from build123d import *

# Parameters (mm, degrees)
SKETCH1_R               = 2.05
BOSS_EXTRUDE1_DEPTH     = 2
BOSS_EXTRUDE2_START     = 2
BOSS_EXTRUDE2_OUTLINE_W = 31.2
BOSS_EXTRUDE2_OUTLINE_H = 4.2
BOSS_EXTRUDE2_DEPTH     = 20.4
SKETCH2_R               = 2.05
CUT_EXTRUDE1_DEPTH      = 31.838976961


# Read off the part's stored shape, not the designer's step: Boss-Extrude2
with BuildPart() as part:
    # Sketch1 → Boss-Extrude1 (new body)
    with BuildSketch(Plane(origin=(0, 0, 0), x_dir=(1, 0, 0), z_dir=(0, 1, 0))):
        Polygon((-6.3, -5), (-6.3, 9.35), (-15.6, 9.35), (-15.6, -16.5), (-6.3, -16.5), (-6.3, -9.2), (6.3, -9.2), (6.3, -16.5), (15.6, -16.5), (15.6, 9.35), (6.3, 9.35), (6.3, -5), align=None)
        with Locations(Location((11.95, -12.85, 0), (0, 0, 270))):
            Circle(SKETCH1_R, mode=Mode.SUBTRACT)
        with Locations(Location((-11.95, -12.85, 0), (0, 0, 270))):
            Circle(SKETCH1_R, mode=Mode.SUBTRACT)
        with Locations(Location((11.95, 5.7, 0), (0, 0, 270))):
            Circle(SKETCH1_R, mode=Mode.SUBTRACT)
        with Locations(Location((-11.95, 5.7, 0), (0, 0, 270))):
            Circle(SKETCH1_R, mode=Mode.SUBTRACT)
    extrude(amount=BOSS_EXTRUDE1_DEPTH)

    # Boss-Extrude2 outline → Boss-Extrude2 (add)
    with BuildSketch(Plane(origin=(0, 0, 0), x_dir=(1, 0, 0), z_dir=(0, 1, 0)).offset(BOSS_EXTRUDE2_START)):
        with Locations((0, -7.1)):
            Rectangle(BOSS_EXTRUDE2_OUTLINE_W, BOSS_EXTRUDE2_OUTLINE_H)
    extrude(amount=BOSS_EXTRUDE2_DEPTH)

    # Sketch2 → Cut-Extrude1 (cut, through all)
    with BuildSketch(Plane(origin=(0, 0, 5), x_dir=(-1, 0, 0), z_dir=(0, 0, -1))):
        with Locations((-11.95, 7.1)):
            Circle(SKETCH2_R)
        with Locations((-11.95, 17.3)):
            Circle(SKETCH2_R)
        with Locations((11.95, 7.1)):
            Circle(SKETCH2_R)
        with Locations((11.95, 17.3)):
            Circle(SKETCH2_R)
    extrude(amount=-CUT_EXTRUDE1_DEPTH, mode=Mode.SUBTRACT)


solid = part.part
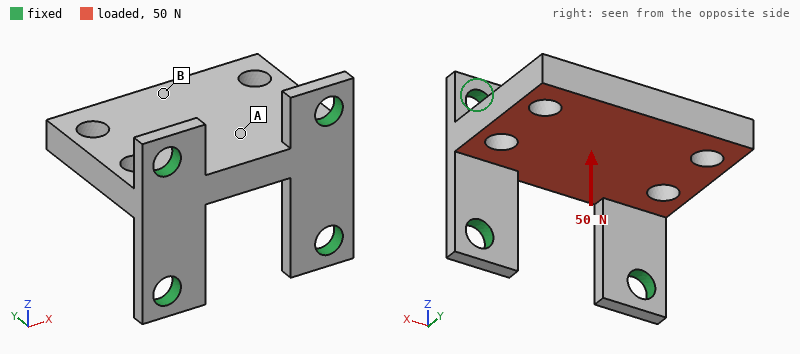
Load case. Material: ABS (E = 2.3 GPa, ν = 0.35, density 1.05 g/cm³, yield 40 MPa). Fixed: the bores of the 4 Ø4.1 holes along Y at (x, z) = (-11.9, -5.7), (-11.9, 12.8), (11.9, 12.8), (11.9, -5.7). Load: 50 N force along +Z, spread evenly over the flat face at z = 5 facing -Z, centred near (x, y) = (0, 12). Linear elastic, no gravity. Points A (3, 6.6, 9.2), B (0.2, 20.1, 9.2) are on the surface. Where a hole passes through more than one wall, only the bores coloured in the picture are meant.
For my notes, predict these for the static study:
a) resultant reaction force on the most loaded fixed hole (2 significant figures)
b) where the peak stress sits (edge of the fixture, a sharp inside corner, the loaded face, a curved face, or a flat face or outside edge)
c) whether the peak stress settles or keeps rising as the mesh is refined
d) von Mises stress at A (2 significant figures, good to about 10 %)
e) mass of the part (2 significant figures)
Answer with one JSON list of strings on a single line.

["27 N", "edge of the fixture", "keeps rising", "2.8 MPa", "3.6 g"]
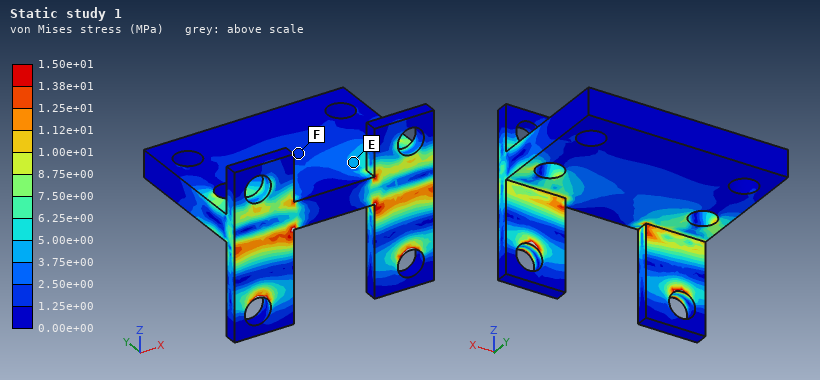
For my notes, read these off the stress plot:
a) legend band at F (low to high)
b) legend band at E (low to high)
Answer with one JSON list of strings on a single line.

["1.25e+00 to 2.50e+00 MPa", "3.75e+00 to 5.00e+00 MPa"]
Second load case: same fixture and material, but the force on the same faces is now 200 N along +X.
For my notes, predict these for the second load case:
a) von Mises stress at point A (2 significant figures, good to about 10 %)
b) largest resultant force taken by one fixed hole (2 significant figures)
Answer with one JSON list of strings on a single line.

["2.4 MPa", "120 N"]
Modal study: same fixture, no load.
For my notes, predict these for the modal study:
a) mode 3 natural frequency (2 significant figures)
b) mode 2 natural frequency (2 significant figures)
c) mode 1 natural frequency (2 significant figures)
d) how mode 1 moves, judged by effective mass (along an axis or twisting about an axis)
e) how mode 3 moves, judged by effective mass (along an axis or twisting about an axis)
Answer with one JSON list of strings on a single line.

["4100 Hz", "3000 Hz", "1200 Hz", "along Z", "along X"]
